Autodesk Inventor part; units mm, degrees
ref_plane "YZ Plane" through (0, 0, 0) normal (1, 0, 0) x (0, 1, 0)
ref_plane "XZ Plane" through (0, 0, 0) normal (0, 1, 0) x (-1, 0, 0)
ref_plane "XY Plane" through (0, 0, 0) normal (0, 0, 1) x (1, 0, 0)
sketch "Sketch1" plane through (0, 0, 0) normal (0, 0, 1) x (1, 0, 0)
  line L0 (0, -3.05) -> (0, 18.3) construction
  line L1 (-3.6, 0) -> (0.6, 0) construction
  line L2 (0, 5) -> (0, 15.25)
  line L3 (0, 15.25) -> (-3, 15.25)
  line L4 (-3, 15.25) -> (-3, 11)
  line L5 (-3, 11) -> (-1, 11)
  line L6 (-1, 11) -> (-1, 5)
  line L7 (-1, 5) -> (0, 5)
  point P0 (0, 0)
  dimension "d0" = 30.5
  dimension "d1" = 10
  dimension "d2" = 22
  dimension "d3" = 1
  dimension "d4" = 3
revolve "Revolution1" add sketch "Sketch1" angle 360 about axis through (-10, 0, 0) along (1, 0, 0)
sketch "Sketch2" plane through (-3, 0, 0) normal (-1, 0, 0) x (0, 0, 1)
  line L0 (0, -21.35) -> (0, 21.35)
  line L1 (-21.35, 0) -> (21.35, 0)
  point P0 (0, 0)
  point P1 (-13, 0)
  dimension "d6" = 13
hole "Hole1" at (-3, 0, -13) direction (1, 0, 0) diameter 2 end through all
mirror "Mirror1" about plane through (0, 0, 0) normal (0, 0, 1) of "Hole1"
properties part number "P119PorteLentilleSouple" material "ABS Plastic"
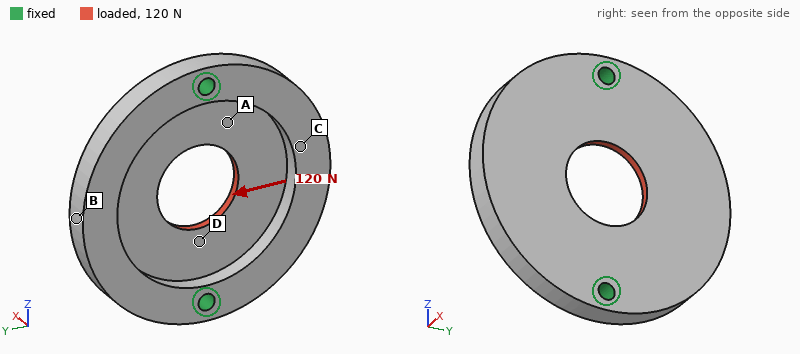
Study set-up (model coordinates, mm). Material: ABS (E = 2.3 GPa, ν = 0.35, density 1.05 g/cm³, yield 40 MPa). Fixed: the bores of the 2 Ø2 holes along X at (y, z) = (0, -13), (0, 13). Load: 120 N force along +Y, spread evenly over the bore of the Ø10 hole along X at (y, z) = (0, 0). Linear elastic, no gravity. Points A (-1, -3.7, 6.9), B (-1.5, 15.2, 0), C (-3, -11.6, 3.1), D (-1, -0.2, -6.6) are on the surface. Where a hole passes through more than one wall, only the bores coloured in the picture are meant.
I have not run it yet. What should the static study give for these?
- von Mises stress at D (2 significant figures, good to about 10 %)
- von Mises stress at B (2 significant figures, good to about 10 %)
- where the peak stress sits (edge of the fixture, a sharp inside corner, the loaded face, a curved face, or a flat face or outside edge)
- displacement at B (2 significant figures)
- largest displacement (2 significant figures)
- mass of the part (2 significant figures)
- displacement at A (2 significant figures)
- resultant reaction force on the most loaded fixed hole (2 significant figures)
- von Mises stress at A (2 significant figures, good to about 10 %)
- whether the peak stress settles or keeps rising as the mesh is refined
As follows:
5.5 MPa
1.6 MPa
edge of the fixture
91 µm
96 µm
1.4 g
22 µm
60 N
4.7 MPa
keeps rising
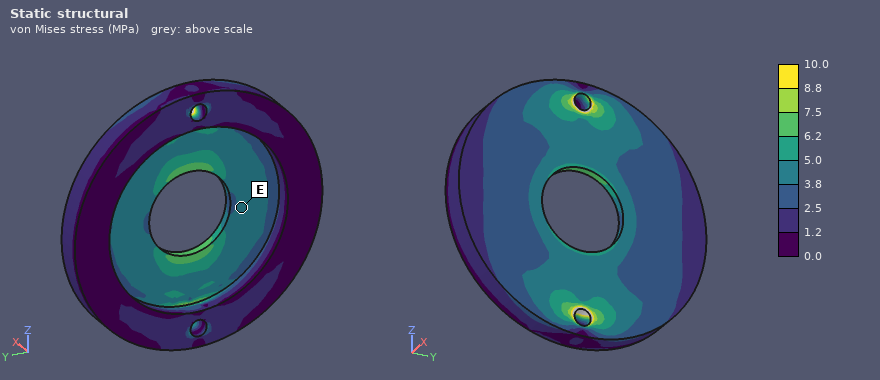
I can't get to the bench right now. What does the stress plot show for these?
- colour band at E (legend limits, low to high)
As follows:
3.8 to 5.0 MPa
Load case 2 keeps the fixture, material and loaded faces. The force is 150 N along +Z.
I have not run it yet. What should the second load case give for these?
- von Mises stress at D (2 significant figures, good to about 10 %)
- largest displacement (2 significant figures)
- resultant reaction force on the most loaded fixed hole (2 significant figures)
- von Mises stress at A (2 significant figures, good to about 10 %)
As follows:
6.6 MPa
40 µm
75 N
6.7 MPa
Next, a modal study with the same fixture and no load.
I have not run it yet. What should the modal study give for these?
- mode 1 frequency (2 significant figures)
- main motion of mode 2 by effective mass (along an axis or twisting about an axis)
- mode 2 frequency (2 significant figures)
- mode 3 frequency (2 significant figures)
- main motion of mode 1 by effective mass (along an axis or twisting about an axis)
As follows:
2200 Hz
along X
2400 Hz
5900 Hz
twisting about Z
